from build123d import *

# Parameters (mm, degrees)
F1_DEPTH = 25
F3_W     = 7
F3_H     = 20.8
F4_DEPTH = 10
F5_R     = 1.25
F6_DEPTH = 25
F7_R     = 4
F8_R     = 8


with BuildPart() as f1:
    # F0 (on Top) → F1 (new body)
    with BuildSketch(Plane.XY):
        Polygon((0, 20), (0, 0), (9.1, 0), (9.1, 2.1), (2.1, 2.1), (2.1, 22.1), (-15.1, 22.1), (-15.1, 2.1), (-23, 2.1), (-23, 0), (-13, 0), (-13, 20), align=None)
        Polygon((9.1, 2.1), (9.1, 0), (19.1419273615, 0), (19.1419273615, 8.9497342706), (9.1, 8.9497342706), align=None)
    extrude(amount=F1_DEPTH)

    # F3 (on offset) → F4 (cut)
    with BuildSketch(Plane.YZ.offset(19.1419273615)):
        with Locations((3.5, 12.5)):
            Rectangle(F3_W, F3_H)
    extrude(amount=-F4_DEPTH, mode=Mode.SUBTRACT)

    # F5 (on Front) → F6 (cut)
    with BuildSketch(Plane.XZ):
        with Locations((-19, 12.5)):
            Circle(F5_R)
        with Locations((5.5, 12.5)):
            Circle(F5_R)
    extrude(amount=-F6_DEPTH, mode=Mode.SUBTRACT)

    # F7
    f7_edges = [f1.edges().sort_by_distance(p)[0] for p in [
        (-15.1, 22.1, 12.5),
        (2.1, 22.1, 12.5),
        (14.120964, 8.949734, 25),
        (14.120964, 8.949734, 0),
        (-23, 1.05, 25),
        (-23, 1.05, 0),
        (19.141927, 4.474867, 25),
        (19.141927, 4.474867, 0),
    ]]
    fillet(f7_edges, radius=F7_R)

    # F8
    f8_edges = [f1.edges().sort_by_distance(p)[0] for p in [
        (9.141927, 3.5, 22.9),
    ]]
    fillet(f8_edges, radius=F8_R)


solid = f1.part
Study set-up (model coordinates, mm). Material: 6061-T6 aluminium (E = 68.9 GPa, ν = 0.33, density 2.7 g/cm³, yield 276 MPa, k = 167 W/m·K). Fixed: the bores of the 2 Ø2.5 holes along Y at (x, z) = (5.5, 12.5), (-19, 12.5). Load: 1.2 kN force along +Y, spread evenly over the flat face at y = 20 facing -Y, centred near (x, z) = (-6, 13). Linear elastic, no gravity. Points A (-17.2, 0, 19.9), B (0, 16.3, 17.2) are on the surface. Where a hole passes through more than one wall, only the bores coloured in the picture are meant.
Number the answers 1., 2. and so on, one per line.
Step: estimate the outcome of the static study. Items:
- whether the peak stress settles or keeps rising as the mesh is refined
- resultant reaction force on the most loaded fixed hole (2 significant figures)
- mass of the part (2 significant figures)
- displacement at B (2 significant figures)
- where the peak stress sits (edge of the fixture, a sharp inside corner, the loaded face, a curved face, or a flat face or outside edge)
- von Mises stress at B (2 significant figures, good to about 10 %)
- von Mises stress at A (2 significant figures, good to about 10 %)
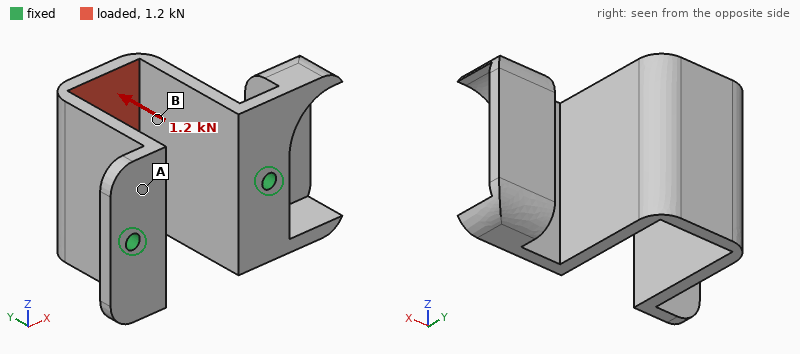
1. keeps rising
2. 610 N
3. 12 g
4. 20 µm
5. edge of the fixture
6. 43 MPa
7. 16 MPa
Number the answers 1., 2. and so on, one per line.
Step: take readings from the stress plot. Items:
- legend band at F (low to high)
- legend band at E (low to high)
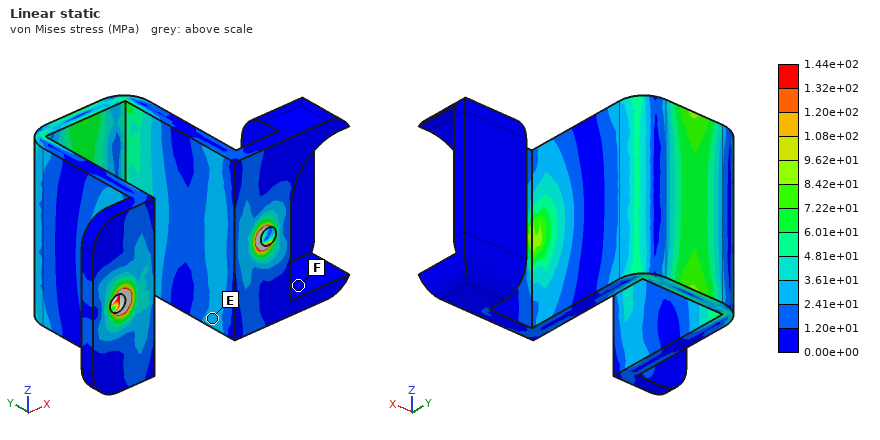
1. 0.00e+00 to 1.20e+01 MPa
2. 2.41e+01 to 3.61e+01 MPa
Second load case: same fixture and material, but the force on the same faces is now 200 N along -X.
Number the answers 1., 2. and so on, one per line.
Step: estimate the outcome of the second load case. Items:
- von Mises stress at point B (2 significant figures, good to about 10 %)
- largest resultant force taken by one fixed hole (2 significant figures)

1. 30 MPa
2. 160 N
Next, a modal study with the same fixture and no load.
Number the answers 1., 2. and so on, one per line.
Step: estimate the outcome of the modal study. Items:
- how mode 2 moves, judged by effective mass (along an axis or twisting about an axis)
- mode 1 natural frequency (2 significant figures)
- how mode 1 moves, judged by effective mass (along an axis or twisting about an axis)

1. along X
2. 2900 Hz
3. along Z
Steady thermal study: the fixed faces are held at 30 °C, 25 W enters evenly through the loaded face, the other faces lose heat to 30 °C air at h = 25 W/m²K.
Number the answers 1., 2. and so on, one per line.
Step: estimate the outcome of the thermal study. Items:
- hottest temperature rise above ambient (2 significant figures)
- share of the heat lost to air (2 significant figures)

1. 44 K
2. 8.7 %
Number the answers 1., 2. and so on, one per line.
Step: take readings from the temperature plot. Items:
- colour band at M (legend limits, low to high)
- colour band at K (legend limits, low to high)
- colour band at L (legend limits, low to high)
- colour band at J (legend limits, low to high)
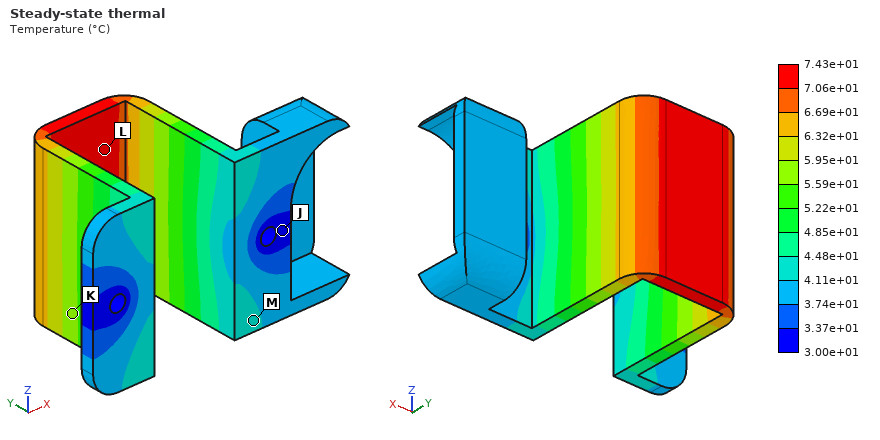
1. 4.11e+01 to 4.48e+01 °C
2. 5.59e+01 to 5.95e+01 °C
3. 7.06e+01 to 7.43e+01 °C
4. 3.00e+01 to 3.37e+01 °C
